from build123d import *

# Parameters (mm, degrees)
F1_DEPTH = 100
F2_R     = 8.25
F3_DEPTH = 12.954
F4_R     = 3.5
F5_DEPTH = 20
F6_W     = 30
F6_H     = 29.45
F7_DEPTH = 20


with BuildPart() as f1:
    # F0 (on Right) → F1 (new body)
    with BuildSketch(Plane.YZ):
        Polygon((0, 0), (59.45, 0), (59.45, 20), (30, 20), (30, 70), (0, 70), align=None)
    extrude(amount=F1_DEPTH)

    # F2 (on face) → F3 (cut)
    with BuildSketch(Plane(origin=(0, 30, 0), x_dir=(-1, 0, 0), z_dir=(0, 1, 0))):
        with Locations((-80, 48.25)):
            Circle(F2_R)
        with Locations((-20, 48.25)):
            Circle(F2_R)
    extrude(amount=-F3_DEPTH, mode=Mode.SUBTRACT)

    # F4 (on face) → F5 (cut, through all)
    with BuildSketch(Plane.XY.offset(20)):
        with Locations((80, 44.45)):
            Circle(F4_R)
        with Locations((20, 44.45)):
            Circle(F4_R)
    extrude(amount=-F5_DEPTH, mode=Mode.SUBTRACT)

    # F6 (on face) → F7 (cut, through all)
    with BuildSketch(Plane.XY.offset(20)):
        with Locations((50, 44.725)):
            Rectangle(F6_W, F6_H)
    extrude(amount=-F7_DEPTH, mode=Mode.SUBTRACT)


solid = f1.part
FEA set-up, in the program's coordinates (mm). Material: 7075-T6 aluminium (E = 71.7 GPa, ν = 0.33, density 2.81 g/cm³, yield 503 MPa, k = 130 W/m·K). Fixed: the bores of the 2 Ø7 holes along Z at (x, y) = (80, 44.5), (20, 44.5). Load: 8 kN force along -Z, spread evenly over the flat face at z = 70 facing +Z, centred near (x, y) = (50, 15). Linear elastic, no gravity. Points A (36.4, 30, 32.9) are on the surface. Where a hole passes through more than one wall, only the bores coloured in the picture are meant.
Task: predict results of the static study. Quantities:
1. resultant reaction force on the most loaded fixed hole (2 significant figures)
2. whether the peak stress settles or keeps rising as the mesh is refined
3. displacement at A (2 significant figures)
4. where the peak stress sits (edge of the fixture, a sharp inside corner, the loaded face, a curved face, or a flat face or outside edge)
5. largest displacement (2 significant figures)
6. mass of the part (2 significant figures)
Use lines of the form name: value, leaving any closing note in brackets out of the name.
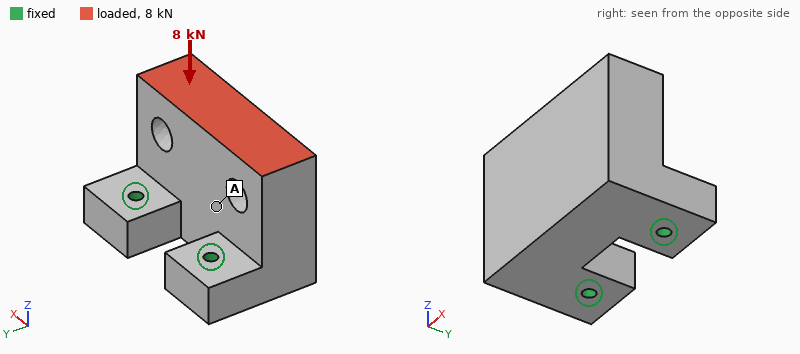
resultant reaction force on the most loaded fixed hole: 4.0 kN
whether the peak stress settles or keeps rising as the mesh is refined: keeps rising
displacement at A: 32 µm
where the peak stress sits: edge of the fixture
largest displacement: 93 µm
mass of the part: 690 g
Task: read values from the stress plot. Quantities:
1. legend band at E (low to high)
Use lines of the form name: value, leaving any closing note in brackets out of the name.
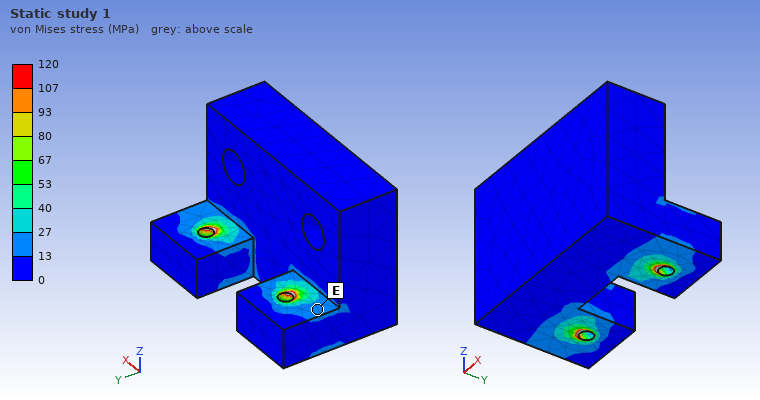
legend band at E: 13 to 27 MPa
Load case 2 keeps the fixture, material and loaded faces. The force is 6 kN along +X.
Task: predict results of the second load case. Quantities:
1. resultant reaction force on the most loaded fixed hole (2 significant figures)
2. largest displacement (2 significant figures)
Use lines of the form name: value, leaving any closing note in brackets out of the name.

resultant reaction force on the most loaded fixed hole: 6.2 kN
largest displacement: 50 µm
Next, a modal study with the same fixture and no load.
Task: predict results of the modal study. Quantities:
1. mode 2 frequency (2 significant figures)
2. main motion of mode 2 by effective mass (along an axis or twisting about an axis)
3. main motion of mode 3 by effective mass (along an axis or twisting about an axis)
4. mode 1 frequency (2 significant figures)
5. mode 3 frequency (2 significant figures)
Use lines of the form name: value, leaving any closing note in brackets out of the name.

mode 2 frequency: 3800 Hz
main motion of mode 2 by effective mass: along X
main motion of mode 3 by effective mass: along X
mode 1 frequency: 1900 Hz
mode 3 frequency: 5600 Hz
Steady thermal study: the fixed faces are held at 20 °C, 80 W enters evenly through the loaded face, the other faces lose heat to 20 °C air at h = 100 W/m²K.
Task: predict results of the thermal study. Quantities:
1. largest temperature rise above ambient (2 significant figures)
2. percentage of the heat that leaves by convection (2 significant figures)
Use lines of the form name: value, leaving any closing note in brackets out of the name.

largest temperature rise above ambient: 18 K
percentage of the heat that leaves by convection: 31 %
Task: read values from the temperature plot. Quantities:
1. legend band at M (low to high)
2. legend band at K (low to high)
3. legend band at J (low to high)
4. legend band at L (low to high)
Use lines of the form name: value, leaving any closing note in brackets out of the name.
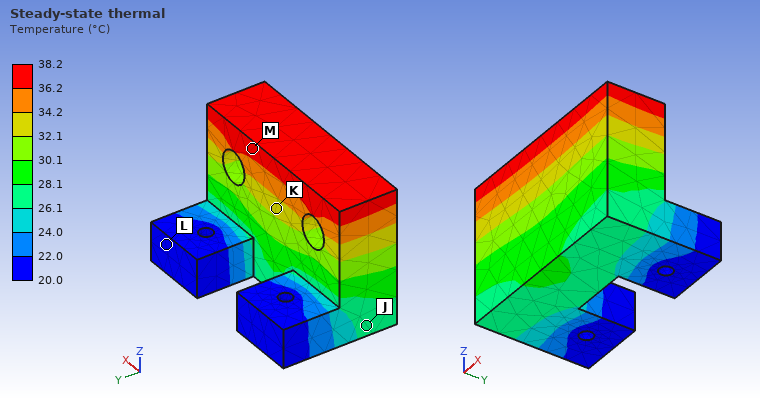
legend band at M: 36.2 to 38.2 °C
legend band at K: 32.1 to 34.2 °C
legend band at J: 26.1 to 28.1 °C
legend band at L: 20.0 to 22.0 °C
